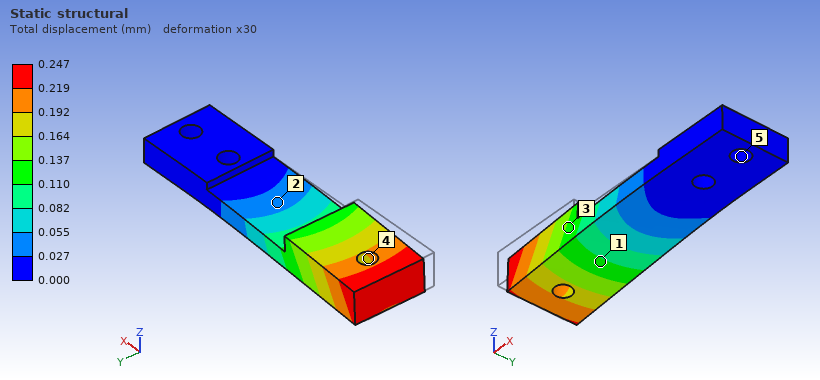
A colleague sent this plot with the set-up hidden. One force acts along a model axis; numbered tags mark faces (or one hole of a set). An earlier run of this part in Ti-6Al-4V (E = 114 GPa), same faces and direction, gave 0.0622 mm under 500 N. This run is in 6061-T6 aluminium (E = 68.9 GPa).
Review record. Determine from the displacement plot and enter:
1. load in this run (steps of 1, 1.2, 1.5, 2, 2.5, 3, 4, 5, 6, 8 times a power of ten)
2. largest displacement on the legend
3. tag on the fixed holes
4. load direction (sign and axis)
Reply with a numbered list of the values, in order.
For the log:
1. 1.2 kN
2. 0.247 mm
3. 5
4. +Y
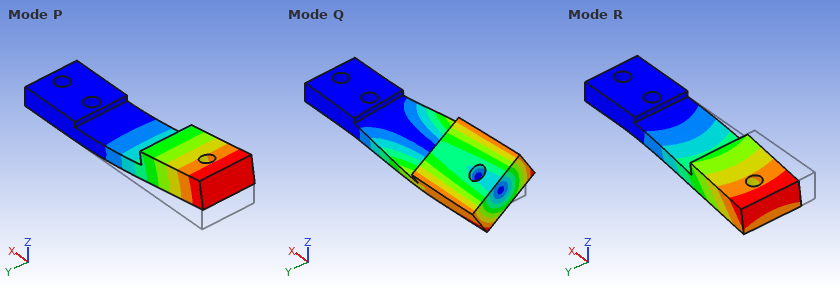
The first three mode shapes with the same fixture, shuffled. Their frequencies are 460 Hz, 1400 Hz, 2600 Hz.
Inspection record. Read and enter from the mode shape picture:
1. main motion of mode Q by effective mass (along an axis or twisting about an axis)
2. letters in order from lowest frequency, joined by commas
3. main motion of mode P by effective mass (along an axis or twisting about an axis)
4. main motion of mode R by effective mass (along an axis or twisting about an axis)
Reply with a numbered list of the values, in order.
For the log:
1. twisting about X
2. P, R, Q
3. along Z
4. along Y
